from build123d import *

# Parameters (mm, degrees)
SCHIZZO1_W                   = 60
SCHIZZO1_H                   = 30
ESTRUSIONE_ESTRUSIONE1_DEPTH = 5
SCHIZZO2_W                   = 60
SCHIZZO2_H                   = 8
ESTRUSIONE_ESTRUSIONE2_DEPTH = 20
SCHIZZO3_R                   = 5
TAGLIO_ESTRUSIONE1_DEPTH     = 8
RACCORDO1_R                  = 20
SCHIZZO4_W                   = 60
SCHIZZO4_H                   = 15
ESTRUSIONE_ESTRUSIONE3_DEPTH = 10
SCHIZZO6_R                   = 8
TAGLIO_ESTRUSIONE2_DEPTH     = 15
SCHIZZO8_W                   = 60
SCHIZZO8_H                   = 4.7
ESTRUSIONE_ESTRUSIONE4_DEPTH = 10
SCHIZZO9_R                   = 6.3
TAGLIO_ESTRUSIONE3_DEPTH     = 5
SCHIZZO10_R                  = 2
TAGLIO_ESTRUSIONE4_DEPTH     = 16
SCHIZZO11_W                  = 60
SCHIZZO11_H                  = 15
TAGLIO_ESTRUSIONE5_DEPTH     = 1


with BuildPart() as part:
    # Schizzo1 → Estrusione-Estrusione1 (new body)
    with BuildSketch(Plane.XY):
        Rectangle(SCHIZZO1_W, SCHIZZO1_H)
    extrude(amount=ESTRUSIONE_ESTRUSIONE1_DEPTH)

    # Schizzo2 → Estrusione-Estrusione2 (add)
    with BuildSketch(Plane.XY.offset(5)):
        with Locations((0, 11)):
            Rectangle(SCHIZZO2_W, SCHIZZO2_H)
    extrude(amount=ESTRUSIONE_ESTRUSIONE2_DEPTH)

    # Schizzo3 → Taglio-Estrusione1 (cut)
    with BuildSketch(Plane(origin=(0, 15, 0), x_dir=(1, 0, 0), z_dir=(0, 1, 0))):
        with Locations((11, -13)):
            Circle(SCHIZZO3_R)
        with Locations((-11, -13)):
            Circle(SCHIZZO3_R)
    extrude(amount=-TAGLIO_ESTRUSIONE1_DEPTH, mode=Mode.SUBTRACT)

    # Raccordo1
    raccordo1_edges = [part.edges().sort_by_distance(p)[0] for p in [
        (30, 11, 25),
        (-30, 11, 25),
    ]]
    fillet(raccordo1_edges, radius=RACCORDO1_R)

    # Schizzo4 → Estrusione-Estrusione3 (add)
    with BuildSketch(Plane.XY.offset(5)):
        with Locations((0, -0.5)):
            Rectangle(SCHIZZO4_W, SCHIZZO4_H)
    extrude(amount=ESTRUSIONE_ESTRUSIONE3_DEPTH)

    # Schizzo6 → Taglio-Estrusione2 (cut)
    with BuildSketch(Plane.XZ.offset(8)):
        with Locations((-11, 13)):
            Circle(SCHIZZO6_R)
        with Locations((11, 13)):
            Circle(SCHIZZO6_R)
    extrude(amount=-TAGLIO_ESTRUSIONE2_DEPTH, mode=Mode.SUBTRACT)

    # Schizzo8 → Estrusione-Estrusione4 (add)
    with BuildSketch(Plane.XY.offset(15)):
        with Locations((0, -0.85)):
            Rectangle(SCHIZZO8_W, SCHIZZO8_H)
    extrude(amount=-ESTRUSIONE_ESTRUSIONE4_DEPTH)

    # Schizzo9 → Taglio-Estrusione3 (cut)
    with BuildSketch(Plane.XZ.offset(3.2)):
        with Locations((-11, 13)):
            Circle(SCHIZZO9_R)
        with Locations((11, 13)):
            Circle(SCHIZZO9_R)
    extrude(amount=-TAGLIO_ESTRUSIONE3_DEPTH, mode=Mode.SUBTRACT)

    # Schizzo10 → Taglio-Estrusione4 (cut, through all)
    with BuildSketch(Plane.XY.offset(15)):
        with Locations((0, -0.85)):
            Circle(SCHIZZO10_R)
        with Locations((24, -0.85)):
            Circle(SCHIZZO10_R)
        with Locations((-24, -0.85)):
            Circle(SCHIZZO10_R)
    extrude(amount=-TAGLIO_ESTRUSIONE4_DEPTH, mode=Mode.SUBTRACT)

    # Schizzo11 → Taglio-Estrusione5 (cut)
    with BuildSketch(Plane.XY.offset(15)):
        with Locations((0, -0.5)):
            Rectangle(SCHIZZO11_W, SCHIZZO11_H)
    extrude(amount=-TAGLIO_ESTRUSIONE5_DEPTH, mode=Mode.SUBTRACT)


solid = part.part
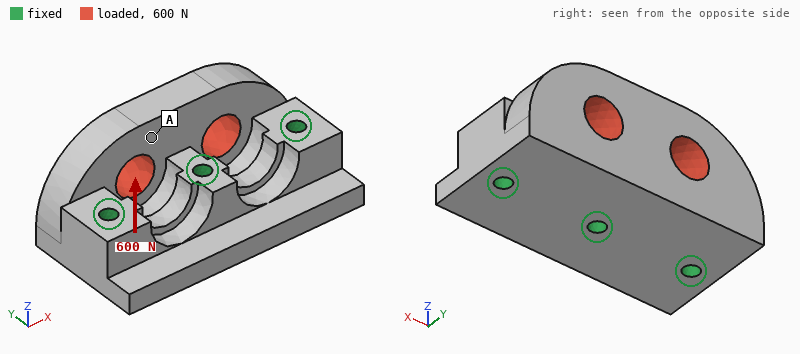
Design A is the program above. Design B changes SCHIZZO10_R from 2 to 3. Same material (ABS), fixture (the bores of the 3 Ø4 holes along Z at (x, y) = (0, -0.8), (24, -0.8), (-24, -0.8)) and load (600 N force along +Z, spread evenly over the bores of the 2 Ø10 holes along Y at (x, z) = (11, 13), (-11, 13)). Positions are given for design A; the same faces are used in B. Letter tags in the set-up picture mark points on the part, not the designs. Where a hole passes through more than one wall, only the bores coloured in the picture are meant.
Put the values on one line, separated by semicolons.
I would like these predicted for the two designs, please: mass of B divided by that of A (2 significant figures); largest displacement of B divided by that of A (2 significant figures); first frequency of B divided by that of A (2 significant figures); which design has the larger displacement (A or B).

0.97; 0.82; 1.1; A
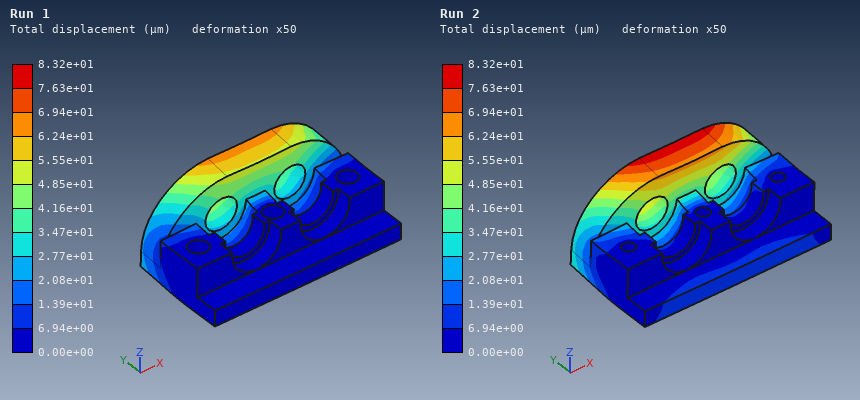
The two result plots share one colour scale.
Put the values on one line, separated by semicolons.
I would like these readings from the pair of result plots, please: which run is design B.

Run 1
